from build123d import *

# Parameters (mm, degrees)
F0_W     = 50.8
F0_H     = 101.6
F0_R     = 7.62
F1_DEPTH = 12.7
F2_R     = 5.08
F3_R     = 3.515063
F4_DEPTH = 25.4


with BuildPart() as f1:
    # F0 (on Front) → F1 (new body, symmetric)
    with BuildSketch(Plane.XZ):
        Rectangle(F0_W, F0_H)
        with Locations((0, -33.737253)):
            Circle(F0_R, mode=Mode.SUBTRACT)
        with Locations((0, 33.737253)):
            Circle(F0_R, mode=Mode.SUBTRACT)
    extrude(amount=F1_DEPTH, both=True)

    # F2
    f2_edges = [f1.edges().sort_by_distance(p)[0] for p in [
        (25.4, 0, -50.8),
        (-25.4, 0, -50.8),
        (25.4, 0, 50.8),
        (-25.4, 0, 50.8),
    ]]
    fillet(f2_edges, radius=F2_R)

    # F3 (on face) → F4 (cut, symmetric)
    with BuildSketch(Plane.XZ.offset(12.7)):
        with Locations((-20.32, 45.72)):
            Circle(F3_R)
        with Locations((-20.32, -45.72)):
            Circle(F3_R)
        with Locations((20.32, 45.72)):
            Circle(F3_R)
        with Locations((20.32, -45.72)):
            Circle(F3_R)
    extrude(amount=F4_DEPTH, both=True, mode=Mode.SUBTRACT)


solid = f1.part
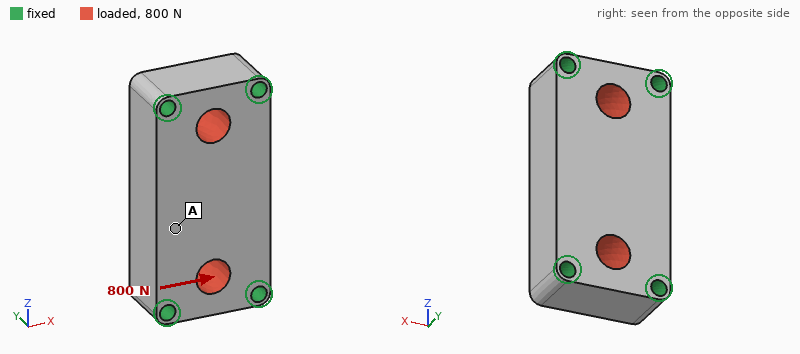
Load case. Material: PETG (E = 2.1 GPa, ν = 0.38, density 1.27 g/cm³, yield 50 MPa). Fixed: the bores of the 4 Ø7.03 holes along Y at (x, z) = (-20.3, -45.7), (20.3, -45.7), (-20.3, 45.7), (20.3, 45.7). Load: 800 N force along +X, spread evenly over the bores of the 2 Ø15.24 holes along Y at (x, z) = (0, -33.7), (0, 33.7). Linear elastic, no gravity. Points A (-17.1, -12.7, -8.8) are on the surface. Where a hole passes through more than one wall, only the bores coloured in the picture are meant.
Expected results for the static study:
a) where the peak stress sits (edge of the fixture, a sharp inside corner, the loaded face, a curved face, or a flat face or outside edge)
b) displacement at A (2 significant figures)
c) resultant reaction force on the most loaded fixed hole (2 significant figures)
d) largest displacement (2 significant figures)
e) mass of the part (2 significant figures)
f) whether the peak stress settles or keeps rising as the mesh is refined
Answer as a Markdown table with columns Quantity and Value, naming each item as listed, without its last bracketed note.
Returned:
| Quantity | Value |
|---|---|
| where the peak stress sits | edge of the fixture |
| displacement at A | 10.0 µm |
| resultant reaction force on the most loaded fixed hole | 220 N |
| largest displacement | 11 µm |
| mass of the part | 150 g |
| whether the peak stress settles or keeps rising as the mesh is refined | keeps rising |
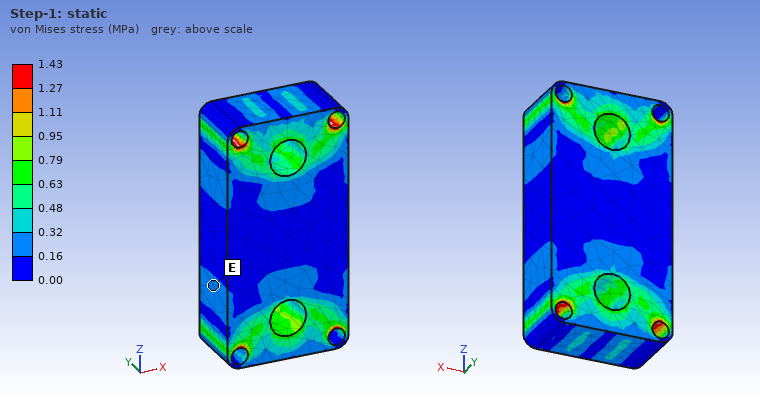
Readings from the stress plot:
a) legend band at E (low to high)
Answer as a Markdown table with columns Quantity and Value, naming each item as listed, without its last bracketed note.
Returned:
| Quantity | Value |
|---|---|
| legend band at E | 0.16 to 0.32 MPa |
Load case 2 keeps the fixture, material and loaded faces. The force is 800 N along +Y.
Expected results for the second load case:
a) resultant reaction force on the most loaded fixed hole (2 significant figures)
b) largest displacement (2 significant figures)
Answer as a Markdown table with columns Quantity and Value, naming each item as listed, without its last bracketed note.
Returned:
| Quantity | Value |
|---|---|
| resultant reaction force on the most loaded fixed hole | 200 N |
| largest displacement | 17 µm |
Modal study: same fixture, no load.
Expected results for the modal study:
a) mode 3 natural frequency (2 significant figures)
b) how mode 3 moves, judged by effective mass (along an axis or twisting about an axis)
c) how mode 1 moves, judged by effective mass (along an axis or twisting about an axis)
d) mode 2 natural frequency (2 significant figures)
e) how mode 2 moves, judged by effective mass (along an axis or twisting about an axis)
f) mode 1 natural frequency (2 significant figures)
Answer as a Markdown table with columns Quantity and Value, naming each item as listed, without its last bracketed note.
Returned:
| Quantity | Value |
|---|---|
| mode 3 natural frequency | 3400 Hz |
| how mode 3 moves, judged by effective mass | twisting about Z |
| how mode 1 moves, judged by effective mass | along Y |
| mode 2 natural frequency | 3000 Hz |
| how mode 2 moves, judged by effective mass | along X |
| mode 1 natural frequency | 2500 Hz |
